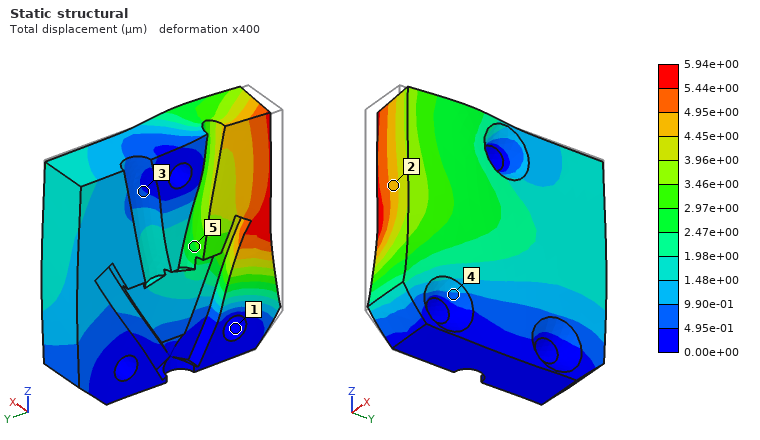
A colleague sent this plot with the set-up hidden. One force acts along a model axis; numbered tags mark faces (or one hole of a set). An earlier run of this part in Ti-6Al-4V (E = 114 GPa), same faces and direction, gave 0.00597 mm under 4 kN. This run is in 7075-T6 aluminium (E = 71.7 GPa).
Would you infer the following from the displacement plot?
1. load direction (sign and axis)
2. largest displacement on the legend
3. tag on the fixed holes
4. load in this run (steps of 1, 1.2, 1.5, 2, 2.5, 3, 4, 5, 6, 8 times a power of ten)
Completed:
+Y
5.94e+00 µm
1
2.5 kN
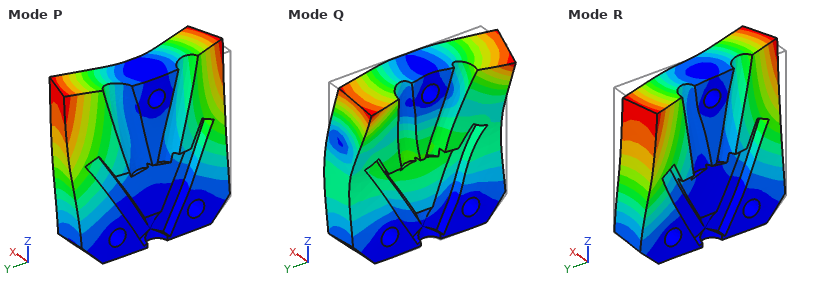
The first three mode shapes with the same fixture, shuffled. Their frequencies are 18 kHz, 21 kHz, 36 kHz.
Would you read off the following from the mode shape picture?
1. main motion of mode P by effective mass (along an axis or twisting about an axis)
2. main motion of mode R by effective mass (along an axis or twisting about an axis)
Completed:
along X
twisting about Z
